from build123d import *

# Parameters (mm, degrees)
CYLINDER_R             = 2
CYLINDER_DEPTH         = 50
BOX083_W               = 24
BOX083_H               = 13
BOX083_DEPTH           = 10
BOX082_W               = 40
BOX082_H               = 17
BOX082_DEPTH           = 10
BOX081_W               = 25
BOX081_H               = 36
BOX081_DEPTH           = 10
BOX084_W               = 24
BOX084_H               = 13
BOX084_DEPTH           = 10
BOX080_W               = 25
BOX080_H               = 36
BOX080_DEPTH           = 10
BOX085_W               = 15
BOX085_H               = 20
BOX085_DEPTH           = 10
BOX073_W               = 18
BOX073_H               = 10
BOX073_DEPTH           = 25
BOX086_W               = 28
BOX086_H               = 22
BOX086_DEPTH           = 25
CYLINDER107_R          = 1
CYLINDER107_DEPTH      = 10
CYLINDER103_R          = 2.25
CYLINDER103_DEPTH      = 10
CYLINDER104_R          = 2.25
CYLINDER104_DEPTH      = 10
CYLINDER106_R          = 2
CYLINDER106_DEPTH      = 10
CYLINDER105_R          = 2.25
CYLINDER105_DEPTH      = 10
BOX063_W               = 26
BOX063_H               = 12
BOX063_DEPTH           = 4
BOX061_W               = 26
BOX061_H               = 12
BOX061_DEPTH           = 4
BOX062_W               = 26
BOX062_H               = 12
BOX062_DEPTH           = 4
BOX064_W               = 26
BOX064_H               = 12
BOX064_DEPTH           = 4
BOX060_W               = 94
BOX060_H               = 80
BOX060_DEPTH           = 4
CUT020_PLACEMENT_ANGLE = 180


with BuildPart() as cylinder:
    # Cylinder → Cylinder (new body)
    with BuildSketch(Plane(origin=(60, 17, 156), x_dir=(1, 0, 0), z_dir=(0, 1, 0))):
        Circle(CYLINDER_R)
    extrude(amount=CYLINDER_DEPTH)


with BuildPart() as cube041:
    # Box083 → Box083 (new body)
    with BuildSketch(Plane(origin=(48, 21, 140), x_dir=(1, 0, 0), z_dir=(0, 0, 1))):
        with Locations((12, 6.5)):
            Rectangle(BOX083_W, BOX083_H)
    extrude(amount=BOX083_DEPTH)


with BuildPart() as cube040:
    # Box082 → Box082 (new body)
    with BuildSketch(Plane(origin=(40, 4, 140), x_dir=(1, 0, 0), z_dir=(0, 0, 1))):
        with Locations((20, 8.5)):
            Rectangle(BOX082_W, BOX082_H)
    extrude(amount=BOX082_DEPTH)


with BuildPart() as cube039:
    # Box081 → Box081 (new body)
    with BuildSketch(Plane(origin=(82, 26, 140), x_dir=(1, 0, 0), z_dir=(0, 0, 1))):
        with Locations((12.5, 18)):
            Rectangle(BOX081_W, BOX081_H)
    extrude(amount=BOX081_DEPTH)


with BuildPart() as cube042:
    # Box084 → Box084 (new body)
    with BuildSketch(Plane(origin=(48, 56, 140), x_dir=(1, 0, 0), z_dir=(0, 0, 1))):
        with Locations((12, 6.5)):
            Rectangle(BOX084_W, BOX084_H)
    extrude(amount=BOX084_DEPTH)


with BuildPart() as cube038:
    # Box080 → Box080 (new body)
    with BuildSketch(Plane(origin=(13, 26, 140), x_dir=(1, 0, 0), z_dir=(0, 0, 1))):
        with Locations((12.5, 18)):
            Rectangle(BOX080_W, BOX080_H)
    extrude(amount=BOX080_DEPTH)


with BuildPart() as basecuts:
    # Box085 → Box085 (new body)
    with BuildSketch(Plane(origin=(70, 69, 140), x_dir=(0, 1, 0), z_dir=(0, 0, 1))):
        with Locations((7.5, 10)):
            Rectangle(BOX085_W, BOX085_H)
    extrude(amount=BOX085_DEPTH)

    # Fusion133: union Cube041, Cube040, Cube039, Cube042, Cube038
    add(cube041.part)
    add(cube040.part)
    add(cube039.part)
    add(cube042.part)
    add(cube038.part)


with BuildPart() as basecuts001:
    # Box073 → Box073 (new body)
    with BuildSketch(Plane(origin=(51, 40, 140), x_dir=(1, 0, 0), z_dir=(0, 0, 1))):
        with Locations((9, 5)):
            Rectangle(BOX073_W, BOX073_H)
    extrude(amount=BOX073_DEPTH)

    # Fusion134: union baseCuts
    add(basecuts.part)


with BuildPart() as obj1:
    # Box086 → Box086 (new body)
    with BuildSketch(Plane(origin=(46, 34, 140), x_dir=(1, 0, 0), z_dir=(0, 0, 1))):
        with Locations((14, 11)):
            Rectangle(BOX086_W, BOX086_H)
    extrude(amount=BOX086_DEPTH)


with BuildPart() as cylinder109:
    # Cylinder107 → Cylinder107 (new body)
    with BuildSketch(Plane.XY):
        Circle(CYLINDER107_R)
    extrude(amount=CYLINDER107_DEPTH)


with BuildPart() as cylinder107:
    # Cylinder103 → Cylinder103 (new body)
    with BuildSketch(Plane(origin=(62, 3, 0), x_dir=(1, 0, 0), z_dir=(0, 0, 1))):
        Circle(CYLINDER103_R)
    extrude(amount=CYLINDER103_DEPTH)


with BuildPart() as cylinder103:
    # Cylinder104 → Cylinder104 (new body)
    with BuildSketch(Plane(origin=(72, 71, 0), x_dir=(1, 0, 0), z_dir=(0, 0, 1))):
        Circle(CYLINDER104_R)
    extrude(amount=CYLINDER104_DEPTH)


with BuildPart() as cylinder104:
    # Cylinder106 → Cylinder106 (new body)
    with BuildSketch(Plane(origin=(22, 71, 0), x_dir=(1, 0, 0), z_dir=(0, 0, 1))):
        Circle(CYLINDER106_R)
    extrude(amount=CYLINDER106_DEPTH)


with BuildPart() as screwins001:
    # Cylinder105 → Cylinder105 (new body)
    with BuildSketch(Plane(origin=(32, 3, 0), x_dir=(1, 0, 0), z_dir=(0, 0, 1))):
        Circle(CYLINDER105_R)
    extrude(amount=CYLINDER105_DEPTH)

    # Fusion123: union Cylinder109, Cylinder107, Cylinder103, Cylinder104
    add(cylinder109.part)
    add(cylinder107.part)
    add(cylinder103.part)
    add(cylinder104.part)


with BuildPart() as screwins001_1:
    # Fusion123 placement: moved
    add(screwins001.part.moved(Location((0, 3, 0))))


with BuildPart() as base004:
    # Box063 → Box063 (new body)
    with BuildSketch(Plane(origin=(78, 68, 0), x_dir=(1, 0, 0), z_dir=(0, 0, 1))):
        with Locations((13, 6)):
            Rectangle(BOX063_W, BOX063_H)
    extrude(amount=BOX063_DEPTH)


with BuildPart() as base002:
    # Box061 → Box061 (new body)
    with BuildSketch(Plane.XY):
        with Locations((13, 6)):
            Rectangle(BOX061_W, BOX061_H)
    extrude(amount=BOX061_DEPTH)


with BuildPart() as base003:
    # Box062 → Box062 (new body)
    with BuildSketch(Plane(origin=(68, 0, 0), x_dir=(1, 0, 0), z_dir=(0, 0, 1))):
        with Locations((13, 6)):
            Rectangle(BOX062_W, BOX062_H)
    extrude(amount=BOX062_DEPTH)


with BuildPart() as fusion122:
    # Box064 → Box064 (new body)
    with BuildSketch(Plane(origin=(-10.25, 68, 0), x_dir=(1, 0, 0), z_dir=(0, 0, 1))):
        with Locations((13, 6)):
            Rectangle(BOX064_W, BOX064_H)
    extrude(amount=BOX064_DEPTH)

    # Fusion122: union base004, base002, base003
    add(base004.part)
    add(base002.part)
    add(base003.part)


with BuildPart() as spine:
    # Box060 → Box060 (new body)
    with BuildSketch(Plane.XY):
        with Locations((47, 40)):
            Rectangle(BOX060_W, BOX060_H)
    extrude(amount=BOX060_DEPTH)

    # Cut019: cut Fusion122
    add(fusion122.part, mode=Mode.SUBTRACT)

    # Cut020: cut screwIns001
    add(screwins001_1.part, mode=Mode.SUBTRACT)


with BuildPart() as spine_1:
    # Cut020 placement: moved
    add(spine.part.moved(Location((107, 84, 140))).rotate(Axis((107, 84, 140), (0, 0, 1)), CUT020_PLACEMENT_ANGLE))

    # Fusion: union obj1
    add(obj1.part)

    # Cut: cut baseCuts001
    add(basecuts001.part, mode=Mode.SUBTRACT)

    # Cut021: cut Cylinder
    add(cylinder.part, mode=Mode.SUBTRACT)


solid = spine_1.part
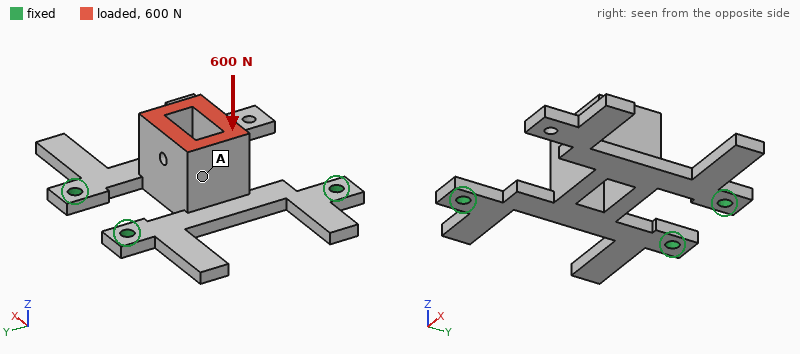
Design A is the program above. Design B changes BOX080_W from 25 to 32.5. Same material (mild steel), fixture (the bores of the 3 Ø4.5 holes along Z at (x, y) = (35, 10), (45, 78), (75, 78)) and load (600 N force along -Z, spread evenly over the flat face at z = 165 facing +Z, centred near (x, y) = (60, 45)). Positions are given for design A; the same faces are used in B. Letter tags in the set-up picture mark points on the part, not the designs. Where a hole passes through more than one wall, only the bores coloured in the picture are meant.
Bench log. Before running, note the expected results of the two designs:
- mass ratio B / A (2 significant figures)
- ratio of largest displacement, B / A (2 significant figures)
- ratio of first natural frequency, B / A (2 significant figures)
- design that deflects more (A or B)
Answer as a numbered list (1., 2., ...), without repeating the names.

1. 0.97
2. 1.1
3. 0.95
4. B
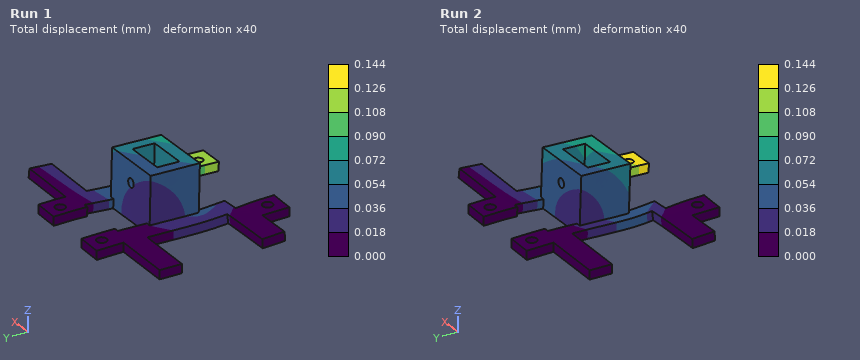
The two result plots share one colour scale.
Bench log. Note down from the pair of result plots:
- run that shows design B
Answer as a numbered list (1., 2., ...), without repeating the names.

1. Run 2
